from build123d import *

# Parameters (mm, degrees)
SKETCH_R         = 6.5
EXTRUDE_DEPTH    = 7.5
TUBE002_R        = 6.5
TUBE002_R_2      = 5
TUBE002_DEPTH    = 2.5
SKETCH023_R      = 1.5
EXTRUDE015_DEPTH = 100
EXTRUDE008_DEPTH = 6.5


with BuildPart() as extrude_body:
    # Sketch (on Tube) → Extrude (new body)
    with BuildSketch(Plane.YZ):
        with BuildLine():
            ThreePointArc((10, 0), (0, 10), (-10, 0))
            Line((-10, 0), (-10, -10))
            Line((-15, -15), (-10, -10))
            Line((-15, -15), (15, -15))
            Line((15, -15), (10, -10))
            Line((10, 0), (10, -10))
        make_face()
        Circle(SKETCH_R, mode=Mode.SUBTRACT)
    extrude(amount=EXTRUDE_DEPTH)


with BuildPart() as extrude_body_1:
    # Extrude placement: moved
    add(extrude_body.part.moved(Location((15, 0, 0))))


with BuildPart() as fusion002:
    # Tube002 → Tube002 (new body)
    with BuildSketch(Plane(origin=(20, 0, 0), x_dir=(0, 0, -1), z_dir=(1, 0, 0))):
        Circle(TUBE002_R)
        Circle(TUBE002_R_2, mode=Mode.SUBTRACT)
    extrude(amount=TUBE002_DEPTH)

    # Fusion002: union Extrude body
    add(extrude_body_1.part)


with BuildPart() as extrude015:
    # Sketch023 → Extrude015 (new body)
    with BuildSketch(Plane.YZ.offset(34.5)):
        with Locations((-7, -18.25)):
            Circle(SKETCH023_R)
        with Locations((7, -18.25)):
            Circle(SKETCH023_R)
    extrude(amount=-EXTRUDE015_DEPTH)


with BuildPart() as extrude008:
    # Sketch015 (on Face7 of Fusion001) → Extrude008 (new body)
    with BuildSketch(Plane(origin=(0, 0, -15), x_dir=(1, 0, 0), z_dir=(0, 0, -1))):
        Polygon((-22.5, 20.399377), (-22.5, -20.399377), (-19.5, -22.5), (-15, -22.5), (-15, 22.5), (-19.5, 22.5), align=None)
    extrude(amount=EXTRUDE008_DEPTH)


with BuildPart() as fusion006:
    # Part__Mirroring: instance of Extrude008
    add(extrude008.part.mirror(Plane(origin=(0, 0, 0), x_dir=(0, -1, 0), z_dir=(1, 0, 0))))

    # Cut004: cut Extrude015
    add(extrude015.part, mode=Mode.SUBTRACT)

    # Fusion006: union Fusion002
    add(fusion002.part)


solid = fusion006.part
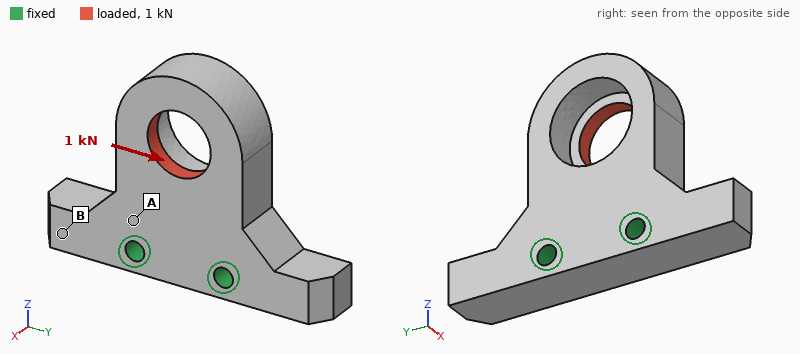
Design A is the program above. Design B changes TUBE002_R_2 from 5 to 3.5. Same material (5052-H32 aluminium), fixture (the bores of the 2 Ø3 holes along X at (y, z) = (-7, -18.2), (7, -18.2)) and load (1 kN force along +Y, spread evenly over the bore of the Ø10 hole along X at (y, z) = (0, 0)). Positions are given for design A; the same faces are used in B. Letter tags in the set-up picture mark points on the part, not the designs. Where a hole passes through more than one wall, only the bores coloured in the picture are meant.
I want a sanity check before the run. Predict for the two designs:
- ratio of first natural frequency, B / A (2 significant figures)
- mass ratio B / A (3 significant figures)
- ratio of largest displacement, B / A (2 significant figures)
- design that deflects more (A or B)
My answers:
0.99
1.02
0.76
A
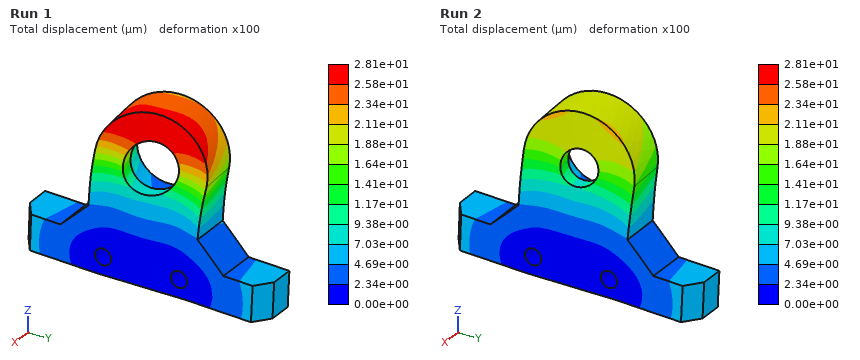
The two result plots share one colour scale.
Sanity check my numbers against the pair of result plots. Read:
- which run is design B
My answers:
Run 2
